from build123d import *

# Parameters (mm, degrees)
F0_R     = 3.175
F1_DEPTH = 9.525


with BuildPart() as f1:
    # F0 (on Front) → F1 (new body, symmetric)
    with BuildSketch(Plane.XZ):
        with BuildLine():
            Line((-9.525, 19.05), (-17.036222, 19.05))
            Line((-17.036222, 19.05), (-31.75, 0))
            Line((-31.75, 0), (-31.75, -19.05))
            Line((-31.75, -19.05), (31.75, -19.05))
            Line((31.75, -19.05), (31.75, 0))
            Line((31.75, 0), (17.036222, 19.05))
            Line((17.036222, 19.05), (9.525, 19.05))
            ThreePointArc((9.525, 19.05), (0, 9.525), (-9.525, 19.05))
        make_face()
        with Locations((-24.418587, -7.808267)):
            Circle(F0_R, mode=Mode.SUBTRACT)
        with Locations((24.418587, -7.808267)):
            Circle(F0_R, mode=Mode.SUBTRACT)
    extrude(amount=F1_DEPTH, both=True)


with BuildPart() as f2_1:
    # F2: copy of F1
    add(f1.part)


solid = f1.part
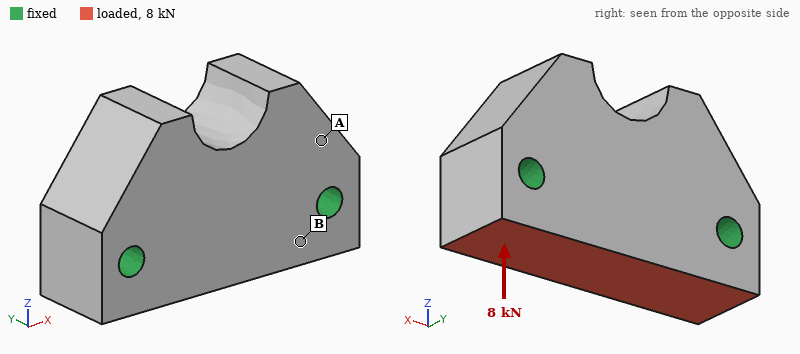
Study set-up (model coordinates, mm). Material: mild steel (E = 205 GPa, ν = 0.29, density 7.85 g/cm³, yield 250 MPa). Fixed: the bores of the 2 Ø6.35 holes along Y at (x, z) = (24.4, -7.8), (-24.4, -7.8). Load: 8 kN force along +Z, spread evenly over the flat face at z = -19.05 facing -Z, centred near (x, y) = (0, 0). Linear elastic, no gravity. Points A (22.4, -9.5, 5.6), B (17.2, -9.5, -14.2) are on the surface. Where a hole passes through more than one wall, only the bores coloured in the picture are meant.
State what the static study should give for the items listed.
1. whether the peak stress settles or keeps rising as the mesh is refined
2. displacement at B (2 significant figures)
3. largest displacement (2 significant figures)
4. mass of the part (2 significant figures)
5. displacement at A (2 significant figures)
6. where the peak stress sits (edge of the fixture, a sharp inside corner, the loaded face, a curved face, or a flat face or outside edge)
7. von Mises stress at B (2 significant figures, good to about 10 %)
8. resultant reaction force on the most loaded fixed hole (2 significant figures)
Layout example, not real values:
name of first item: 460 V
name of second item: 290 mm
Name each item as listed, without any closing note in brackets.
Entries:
whether the peak stress settles or keeps rising as the mesh is refined: keeps rising
displacement at B: 0.81 µm
largest displacement: 1.8 µm
mass of the part: 290 g
displacement at A: 0.48 µm
where the peak stress sits: edge of the fixture
von Mises stress at B: 9.3 MPa
resultant reaction force on the most loaded fixed hole: 4.0 kN
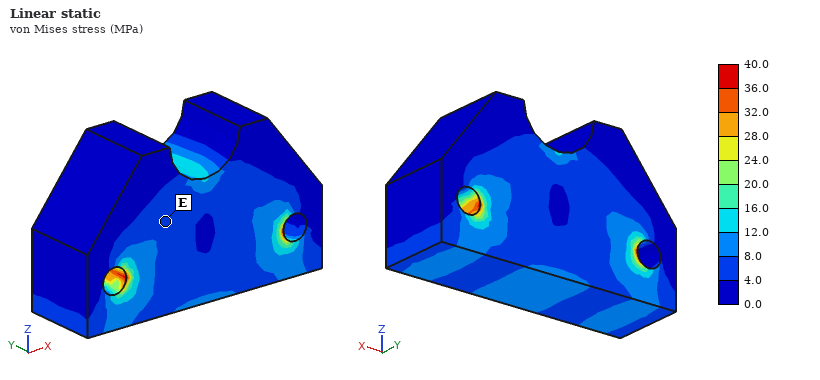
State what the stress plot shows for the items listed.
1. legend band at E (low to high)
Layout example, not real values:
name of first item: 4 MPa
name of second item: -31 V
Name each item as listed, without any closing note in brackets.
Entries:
legend band at E: 4.0 to 8.0 MPa
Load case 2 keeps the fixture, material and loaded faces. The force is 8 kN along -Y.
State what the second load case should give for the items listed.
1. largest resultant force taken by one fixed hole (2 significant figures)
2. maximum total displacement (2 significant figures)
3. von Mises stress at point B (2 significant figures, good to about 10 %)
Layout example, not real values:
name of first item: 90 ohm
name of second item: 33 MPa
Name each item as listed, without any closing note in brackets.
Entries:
largest resultant force taken by one fixed hole: 4.0 kN
maximum total displacement: 5.6 µm
von Mises stress at point B: 20 MPa
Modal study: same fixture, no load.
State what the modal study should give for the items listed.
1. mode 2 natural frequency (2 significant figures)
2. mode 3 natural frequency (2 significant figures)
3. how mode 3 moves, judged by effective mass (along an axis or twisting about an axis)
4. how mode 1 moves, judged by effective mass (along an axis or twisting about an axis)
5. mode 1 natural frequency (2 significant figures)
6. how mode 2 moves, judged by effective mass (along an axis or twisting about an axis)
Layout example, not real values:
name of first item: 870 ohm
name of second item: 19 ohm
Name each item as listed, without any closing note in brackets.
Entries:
mode 2 natural frequency: 21 kHz
mode 3 natural frequency: 25 kHz
how mode 3 moves, judged by effective mass: along Y
how mode 1 moves, judged by effective mass: along Y
mode 1 natural frequency: 16 kHz
how mode 2 moves, judged by effective mass: along Z
